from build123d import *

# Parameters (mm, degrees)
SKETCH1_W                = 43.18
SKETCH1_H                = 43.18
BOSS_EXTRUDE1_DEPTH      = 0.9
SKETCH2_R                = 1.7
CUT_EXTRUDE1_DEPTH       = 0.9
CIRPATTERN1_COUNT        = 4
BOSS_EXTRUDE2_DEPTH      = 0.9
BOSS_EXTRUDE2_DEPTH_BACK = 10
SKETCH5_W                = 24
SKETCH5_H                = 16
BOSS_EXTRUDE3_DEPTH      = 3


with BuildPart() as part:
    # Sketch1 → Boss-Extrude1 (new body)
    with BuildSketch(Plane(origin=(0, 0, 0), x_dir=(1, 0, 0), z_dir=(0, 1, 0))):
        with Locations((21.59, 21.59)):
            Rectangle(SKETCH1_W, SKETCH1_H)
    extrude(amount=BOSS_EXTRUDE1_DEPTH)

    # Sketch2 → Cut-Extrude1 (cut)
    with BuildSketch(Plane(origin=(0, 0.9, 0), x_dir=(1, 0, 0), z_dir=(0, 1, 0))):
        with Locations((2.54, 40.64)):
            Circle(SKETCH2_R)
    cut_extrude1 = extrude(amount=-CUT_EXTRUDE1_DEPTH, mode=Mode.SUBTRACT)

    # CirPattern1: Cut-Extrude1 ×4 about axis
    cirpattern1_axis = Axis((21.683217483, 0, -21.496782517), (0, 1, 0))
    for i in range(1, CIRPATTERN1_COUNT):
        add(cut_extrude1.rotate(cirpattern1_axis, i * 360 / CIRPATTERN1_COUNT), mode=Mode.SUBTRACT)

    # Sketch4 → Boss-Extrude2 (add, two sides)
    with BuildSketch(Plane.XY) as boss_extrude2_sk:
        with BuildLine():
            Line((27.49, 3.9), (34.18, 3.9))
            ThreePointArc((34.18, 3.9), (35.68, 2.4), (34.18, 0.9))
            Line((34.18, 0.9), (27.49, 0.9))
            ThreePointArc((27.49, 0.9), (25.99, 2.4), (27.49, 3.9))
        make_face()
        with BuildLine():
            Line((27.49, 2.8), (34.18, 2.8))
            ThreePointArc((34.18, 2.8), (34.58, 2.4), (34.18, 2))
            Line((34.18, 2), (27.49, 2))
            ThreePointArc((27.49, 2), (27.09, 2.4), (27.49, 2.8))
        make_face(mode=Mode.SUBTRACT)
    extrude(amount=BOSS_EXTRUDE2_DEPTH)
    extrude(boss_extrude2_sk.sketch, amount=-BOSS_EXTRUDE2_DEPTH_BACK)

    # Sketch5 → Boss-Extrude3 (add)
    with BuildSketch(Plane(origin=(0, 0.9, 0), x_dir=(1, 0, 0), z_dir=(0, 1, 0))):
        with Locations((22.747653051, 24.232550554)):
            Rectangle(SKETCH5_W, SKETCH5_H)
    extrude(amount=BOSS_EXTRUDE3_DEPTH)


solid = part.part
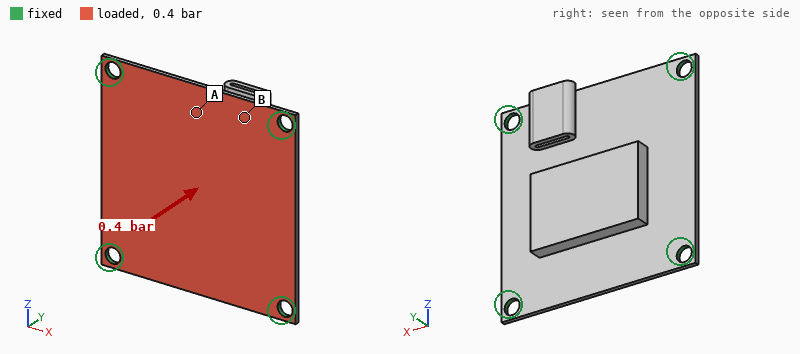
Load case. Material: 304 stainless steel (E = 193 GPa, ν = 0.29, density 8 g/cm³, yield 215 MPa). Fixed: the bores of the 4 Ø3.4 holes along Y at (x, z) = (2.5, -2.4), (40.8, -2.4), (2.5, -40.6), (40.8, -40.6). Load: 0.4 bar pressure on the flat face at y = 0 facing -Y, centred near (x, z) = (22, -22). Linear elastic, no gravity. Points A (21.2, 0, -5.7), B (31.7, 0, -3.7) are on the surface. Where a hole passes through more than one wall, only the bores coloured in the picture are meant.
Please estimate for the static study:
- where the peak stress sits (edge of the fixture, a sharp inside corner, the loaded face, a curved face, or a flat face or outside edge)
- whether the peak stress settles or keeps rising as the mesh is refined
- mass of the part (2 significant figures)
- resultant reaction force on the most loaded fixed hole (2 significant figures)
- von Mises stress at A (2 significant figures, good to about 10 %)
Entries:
edge of the fixture
keeps rising
24 g
21 N
13 MPa
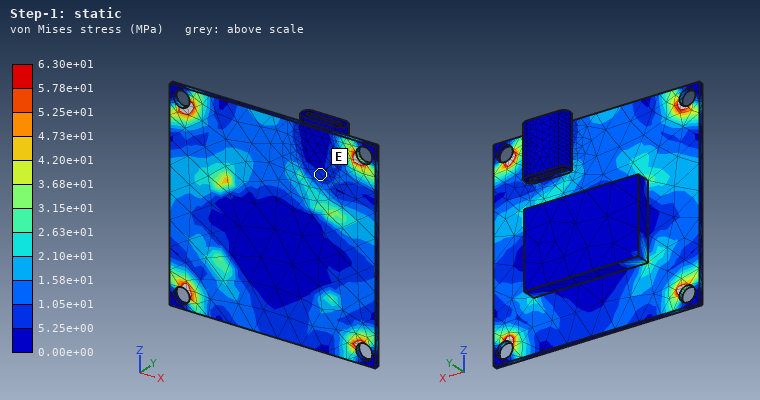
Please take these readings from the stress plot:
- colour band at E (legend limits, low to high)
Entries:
5.25e+00 to 1.05e+01 MPa
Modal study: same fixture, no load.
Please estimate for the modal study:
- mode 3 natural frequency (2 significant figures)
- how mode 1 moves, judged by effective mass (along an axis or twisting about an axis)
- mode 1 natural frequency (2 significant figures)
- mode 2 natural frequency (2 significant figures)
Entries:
4100 Hz
along Y
2100 Hz
4000 Hz
